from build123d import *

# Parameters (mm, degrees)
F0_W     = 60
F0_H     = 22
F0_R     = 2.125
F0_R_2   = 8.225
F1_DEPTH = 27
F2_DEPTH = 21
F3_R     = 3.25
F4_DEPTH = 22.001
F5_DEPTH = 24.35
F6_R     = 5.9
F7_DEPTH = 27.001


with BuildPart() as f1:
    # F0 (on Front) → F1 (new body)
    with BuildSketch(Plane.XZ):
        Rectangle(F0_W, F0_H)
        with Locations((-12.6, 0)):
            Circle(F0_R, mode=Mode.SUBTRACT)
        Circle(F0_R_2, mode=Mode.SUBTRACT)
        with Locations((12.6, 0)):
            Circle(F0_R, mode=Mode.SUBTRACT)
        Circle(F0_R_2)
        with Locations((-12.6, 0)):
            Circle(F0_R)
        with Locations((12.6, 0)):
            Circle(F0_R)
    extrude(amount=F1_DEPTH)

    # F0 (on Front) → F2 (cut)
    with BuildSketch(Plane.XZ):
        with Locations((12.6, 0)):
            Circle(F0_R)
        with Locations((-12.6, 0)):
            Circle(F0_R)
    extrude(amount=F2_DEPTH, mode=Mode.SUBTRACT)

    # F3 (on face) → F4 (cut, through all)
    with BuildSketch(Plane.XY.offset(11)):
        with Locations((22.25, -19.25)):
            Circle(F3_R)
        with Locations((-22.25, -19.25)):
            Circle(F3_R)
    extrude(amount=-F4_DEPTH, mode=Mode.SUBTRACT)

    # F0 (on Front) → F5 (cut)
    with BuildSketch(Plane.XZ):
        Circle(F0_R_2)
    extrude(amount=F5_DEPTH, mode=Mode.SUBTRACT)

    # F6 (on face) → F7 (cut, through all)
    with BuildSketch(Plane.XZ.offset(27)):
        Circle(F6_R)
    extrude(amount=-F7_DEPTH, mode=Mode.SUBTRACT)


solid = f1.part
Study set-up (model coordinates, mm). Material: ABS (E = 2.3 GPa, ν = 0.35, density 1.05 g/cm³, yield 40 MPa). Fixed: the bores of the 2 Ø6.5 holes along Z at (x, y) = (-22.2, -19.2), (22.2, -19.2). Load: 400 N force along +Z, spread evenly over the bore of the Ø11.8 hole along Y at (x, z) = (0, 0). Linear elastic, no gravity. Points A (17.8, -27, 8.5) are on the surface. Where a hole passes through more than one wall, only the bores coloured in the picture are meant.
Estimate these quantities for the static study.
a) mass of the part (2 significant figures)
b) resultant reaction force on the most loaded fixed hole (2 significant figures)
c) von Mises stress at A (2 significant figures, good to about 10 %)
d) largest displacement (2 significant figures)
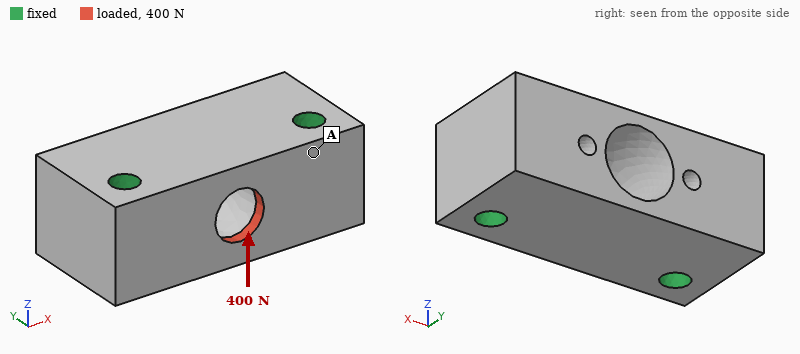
30 g
200 N
1.0 MPa
60 µm
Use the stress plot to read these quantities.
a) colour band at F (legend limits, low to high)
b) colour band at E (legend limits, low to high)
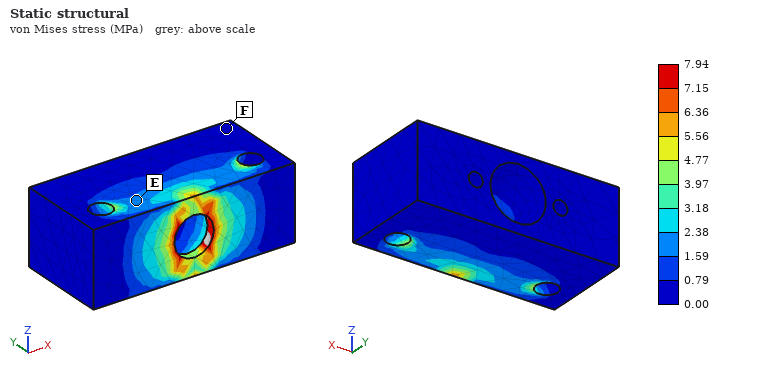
0.00 to 0.79 MPa
1.59 to 2.38 MPa
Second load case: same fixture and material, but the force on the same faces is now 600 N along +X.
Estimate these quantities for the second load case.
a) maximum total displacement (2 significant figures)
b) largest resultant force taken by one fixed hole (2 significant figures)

30 µm
310 N
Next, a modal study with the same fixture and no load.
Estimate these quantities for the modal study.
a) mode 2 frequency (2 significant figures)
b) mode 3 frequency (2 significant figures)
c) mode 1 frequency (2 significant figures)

7000 Hz
8400 Hz
6900 Hz
